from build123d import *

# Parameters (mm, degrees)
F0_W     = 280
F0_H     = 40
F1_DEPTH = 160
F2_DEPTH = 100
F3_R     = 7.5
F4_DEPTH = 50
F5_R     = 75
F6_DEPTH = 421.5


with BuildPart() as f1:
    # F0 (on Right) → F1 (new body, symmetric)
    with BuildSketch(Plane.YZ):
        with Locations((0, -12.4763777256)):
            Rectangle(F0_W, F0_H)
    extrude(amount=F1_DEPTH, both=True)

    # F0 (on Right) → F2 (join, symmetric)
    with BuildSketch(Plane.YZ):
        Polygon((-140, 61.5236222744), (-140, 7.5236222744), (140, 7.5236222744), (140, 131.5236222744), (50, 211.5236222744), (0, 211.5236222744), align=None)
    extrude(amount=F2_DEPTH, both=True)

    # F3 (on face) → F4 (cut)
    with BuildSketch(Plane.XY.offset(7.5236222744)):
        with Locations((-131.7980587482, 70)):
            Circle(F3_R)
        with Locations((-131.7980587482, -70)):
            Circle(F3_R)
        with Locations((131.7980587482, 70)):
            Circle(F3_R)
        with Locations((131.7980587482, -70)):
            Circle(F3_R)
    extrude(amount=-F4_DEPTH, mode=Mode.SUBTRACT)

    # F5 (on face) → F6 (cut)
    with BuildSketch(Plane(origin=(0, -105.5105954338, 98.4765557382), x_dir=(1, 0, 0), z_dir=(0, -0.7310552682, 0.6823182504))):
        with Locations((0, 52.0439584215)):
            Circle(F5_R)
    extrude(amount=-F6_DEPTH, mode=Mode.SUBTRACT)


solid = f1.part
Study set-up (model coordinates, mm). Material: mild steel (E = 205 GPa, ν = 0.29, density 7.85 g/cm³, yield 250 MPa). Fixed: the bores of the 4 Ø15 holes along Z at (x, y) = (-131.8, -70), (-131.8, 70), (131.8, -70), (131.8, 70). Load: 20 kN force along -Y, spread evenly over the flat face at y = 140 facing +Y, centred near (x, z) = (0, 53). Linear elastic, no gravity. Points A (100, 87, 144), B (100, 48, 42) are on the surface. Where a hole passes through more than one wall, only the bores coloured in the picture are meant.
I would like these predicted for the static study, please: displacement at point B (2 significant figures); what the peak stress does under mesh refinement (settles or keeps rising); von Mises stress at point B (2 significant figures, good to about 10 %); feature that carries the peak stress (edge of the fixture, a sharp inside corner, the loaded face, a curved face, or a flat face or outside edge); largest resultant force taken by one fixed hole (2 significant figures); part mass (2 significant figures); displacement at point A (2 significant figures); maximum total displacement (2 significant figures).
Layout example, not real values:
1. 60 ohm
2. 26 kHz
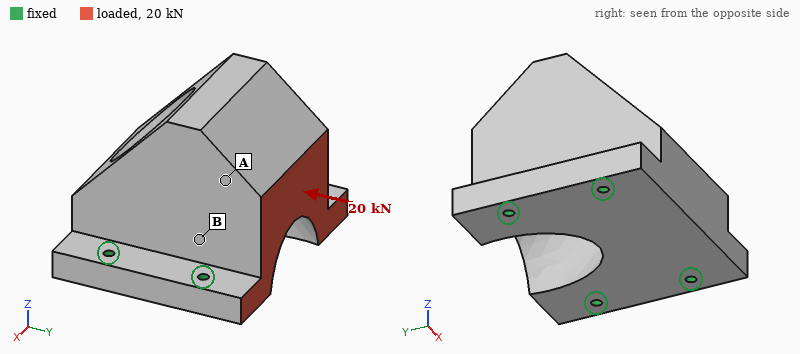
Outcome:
1. 3.1 µm
2. keeps rising
3. 2.6 MPa
4. edge of the fixture
5. 7.2 kN
6. 63 kg
7. 6.3 µm
8. 7.9 µm
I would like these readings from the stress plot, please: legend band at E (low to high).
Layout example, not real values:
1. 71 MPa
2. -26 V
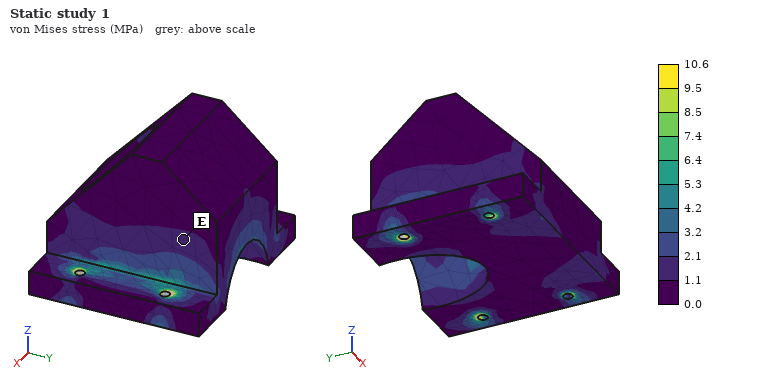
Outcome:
1. 1.1 to 2.1 MPa
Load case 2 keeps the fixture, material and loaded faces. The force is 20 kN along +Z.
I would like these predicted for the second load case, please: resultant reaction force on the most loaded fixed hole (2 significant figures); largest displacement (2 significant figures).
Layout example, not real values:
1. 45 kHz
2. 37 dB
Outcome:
1. 14 kN
2. 12 µm
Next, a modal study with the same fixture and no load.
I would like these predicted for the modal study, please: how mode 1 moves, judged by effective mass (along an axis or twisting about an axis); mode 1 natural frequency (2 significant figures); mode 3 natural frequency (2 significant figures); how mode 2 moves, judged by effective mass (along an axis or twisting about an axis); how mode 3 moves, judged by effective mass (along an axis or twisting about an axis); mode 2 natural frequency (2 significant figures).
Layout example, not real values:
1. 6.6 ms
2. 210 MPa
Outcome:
1. along Y
2. 1100 Hz
3. 2000 Hz
4. along X
5. along Z
6. 1400 Hz
